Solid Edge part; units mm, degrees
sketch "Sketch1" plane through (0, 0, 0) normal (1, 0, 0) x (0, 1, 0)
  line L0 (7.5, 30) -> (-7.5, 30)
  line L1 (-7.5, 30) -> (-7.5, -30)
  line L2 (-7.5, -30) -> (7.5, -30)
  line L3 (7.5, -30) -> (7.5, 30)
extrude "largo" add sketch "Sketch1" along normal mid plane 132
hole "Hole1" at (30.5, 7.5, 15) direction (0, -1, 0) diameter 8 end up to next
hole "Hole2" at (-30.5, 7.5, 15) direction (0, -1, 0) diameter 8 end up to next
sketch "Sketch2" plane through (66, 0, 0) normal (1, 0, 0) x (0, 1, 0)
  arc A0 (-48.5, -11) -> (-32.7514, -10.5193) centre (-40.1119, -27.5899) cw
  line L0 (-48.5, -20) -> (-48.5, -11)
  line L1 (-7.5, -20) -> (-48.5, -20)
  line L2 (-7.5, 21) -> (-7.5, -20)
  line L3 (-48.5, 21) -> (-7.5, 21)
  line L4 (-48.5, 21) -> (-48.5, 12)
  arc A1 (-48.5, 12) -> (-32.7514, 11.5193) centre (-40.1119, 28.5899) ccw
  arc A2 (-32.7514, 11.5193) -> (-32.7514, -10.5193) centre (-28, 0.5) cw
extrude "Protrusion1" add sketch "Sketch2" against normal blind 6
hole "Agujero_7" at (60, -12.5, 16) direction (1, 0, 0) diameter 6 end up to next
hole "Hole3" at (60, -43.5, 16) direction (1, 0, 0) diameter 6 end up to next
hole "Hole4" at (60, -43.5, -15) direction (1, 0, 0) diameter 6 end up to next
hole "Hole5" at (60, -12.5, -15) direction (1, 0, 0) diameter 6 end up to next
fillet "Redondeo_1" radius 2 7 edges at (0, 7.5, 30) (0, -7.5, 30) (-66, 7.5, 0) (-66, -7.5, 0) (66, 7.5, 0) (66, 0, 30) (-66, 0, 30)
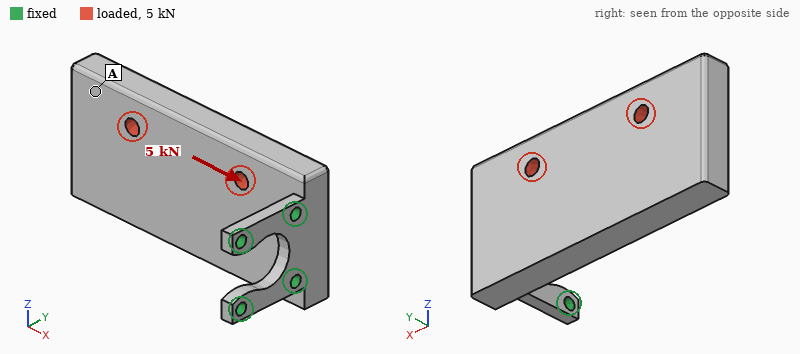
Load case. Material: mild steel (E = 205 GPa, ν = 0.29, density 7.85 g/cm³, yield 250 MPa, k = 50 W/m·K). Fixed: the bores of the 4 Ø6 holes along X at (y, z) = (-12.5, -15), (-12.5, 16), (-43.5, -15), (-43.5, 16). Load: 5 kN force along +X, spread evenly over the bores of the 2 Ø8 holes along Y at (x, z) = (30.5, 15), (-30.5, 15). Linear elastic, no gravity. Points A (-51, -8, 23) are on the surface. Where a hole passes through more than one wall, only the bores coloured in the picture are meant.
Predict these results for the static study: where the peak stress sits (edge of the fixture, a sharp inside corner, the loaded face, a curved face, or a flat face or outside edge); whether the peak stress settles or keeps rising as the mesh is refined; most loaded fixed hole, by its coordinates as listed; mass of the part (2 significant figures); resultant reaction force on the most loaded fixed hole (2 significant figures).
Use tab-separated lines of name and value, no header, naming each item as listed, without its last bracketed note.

where the peak stress sits	edge of the fixture
whether the peak stress settles or keeps rising as the mesh is refined	keeps rising
most loaded fixed hole, by its coordinates as listed	(-12.5, 16)
mass of the part	960 g
resultant reaction force on the most loaded fixed hole	4.8 kN
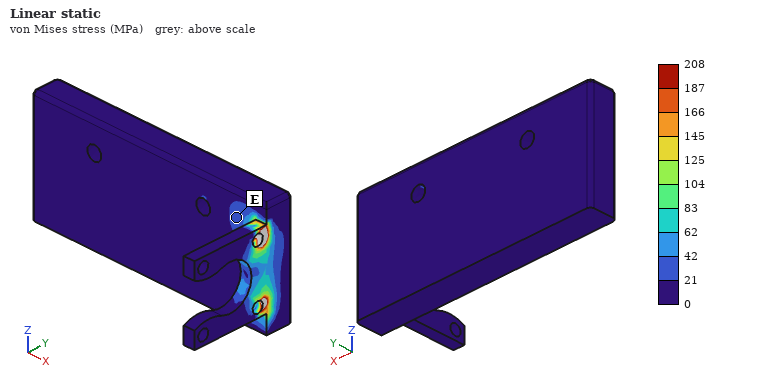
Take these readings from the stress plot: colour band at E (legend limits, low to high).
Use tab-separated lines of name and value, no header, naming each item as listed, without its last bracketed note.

colour band at E	21 to 42 MPa
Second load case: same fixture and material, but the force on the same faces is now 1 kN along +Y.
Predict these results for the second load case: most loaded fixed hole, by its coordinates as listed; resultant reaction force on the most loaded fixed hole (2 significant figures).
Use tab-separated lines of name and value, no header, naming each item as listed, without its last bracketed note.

most loaded fixed hole, by its coordinates as listed	(-12.5, 16)
resultant reaction force on the most loaded fixed hole	990 N
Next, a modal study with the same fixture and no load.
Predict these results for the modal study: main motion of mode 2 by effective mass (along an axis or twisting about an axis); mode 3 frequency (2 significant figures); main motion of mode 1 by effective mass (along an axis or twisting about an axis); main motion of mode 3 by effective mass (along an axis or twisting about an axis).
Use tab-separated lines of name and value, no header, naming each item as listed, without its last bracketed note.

main motion of mode 2 by effective mass	along Z
mode 3 frequency	2700 Hz
main motion of mode 1 by effective mass	along Y
main motion of mode 3 by effective mass	twisting about X
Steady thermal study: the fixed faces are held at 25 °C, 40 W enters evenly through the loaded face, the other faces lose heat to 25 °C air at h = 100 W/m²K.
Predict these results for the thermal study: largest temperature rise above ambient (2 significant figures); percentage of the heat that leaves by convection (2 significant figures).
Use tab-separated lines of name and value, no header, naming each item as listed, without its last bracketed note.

largest temperature rise above ambient	26 K
percentage of the heat that leaves by convection	76 %
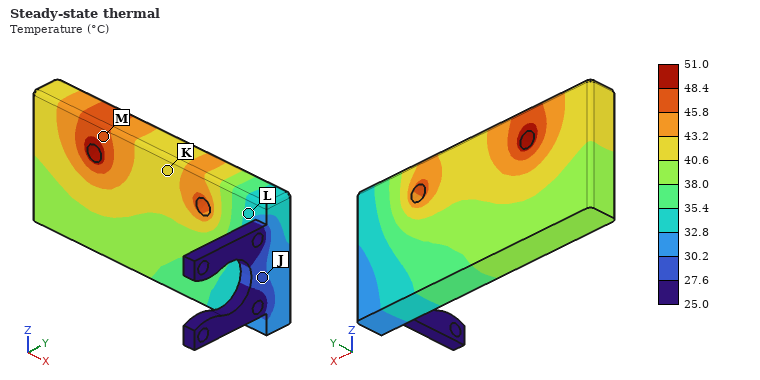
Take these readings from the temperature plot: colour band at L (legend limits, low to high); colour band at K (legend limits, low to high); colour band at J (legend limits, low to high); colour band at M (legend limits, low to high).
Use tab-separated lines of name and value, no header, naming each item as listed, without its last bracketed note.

colour band at L	32.8 to 35.4 °C
colour band at K	40.6 to 43.2 °C
colour band at J	27.6 to 30.2 °C
colour band at M	45.8 to 48.4 °C
